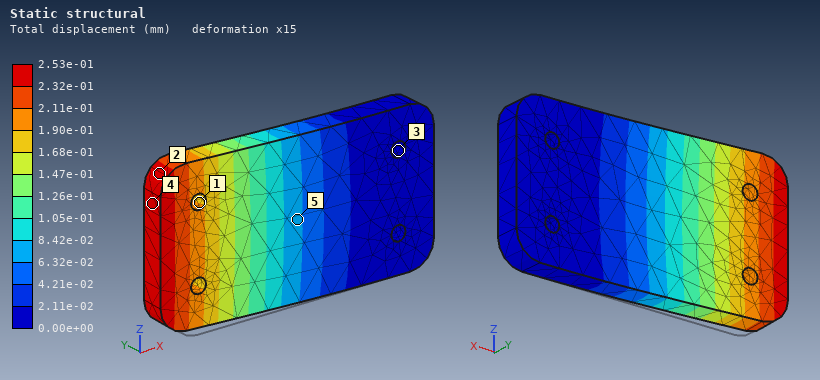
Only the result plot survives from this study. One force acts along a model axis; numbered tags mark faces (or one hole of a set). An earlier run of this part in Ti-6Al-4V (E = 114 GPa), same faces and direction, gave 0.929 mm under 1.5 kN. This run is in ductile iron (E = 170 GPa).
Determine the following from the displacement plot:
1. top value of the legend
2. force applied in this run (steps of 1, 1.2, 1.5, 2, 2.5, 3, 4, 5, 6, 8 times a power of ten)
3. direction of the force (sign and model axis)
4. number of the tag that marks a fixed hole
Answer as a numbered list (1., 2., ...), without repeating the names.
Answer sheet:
1. 2.53e-01 mm
2. 600 N
3. +Y
4. 3
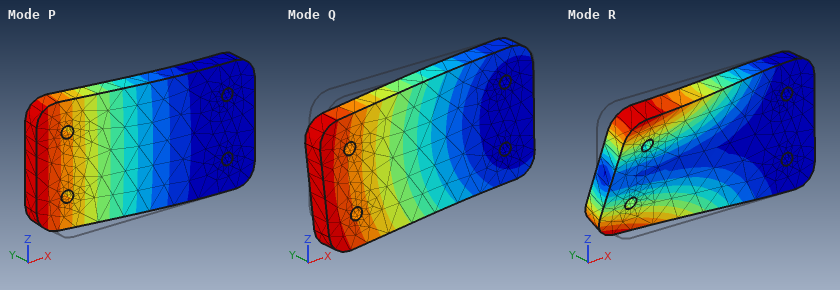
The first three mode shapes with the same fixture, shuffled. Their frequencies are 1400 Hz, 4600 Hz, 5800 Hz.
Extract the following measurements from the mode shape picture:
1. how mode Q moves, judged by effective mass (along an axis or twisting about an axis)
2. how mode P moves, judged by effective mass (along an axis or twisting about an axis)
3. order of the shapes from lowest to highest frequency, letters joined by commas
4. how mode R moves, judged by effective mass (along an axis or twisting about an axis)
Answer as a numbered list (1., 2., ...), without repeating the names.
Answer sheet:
1. along Z
2. along Y
3. P, R, Q
4. twisting about X
